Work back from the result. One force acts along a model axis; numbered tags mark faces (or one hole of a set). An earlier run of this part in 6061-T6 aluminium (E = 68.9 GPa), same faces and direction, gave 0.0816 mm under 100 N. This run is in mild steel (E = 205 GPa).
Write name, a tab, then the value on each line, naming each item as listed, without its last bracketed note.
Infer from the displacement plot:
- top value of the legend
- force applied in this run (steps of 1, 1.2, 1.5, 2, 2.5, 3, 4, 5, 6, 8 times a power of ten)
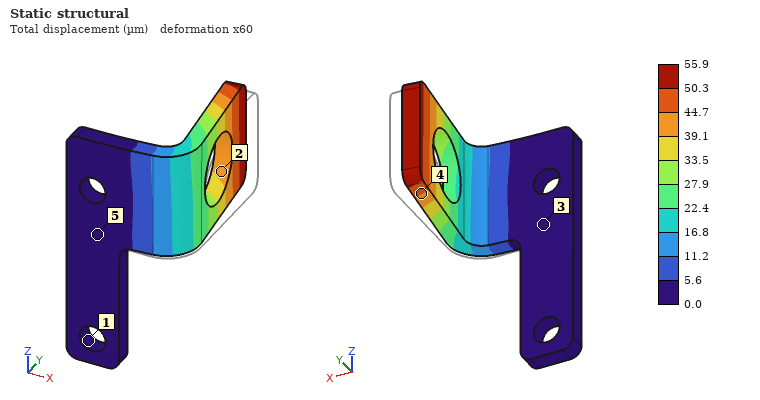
top value of the legend	55.9 µm
force applied in this run	200 N
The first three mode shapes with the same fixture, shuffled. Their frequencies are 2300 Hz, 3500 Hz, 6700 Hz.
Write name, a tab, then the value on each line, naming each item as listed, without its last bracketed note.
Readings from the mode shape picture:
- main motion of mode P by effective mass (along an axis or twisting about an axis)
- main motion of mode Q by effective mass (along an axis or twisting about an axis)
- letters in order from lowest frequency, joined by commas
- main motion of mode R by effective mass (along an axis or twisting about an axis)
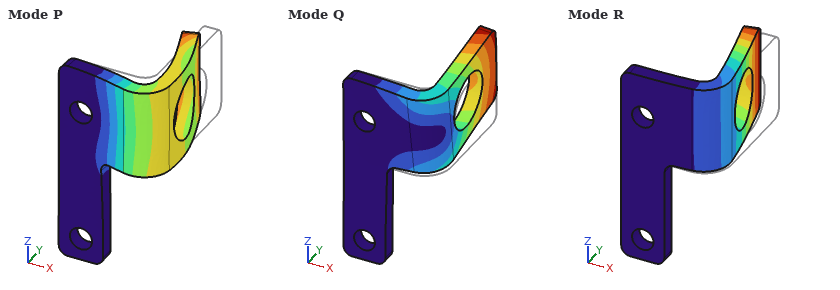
main motion of mode P by effective mass	along Y
main motion of mode Q by effective mass	along Z
letters in order from lowest frequency, joined by commas	R, Q, P
main motion of mode R by effective mass	along X
